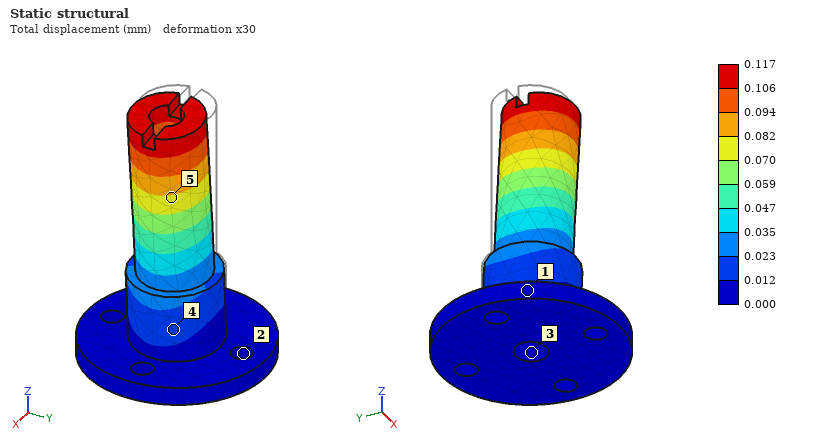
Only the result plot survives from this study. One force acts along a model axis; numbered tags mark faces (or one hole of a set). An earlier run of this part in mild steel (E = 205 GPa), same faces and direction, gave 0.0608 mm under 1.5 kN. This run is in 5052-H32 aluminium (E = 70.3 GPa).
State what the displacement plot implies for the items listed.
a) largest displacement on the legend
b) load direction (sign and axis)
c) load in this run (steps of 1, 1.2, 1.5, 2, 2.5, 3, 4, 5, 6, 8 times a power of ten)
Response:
0.117 mm
+X
1 kN
